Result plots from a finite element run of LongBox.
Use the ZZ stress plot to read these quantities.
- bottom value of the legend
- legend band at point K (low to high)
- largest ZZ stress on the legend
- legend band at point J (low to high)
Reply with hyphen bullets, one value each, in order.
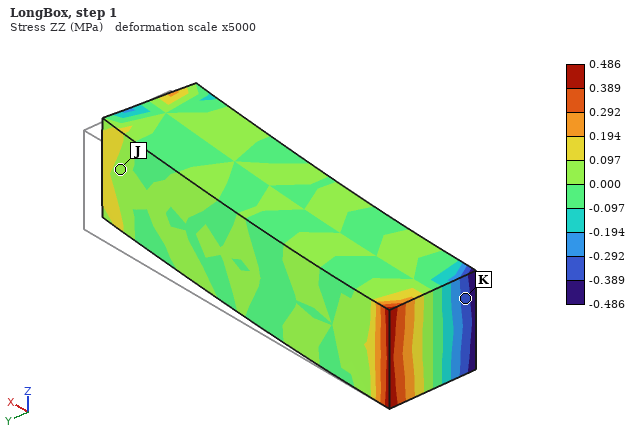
- -0.486 MPa
- -0.389 to -0.292 MPa
- 0.486 MPa
- 0.000 to 0.097 MPa
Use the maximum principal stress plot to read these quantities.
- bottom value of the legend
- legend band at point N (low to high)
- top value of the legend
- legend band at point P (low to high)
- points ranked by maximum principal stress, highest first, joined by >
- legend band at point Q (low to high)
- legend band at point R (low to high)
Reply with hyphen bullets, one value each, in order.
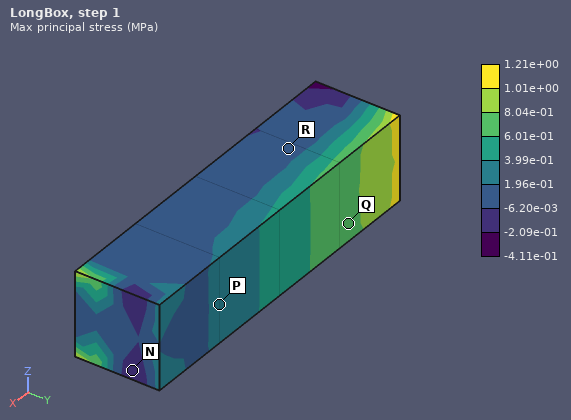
- -4.11e-01 MPa
- -2.09e-01 to -6.20e-03 MPa
- 1.21e+00 MPa
- 1.96e-01 to 3.99e-01 MPa
- Q > P > R > N
- 6.01e-01 to 8.04e-01 MPa
- -6.20e-03 to 1.96e-01 MPa
